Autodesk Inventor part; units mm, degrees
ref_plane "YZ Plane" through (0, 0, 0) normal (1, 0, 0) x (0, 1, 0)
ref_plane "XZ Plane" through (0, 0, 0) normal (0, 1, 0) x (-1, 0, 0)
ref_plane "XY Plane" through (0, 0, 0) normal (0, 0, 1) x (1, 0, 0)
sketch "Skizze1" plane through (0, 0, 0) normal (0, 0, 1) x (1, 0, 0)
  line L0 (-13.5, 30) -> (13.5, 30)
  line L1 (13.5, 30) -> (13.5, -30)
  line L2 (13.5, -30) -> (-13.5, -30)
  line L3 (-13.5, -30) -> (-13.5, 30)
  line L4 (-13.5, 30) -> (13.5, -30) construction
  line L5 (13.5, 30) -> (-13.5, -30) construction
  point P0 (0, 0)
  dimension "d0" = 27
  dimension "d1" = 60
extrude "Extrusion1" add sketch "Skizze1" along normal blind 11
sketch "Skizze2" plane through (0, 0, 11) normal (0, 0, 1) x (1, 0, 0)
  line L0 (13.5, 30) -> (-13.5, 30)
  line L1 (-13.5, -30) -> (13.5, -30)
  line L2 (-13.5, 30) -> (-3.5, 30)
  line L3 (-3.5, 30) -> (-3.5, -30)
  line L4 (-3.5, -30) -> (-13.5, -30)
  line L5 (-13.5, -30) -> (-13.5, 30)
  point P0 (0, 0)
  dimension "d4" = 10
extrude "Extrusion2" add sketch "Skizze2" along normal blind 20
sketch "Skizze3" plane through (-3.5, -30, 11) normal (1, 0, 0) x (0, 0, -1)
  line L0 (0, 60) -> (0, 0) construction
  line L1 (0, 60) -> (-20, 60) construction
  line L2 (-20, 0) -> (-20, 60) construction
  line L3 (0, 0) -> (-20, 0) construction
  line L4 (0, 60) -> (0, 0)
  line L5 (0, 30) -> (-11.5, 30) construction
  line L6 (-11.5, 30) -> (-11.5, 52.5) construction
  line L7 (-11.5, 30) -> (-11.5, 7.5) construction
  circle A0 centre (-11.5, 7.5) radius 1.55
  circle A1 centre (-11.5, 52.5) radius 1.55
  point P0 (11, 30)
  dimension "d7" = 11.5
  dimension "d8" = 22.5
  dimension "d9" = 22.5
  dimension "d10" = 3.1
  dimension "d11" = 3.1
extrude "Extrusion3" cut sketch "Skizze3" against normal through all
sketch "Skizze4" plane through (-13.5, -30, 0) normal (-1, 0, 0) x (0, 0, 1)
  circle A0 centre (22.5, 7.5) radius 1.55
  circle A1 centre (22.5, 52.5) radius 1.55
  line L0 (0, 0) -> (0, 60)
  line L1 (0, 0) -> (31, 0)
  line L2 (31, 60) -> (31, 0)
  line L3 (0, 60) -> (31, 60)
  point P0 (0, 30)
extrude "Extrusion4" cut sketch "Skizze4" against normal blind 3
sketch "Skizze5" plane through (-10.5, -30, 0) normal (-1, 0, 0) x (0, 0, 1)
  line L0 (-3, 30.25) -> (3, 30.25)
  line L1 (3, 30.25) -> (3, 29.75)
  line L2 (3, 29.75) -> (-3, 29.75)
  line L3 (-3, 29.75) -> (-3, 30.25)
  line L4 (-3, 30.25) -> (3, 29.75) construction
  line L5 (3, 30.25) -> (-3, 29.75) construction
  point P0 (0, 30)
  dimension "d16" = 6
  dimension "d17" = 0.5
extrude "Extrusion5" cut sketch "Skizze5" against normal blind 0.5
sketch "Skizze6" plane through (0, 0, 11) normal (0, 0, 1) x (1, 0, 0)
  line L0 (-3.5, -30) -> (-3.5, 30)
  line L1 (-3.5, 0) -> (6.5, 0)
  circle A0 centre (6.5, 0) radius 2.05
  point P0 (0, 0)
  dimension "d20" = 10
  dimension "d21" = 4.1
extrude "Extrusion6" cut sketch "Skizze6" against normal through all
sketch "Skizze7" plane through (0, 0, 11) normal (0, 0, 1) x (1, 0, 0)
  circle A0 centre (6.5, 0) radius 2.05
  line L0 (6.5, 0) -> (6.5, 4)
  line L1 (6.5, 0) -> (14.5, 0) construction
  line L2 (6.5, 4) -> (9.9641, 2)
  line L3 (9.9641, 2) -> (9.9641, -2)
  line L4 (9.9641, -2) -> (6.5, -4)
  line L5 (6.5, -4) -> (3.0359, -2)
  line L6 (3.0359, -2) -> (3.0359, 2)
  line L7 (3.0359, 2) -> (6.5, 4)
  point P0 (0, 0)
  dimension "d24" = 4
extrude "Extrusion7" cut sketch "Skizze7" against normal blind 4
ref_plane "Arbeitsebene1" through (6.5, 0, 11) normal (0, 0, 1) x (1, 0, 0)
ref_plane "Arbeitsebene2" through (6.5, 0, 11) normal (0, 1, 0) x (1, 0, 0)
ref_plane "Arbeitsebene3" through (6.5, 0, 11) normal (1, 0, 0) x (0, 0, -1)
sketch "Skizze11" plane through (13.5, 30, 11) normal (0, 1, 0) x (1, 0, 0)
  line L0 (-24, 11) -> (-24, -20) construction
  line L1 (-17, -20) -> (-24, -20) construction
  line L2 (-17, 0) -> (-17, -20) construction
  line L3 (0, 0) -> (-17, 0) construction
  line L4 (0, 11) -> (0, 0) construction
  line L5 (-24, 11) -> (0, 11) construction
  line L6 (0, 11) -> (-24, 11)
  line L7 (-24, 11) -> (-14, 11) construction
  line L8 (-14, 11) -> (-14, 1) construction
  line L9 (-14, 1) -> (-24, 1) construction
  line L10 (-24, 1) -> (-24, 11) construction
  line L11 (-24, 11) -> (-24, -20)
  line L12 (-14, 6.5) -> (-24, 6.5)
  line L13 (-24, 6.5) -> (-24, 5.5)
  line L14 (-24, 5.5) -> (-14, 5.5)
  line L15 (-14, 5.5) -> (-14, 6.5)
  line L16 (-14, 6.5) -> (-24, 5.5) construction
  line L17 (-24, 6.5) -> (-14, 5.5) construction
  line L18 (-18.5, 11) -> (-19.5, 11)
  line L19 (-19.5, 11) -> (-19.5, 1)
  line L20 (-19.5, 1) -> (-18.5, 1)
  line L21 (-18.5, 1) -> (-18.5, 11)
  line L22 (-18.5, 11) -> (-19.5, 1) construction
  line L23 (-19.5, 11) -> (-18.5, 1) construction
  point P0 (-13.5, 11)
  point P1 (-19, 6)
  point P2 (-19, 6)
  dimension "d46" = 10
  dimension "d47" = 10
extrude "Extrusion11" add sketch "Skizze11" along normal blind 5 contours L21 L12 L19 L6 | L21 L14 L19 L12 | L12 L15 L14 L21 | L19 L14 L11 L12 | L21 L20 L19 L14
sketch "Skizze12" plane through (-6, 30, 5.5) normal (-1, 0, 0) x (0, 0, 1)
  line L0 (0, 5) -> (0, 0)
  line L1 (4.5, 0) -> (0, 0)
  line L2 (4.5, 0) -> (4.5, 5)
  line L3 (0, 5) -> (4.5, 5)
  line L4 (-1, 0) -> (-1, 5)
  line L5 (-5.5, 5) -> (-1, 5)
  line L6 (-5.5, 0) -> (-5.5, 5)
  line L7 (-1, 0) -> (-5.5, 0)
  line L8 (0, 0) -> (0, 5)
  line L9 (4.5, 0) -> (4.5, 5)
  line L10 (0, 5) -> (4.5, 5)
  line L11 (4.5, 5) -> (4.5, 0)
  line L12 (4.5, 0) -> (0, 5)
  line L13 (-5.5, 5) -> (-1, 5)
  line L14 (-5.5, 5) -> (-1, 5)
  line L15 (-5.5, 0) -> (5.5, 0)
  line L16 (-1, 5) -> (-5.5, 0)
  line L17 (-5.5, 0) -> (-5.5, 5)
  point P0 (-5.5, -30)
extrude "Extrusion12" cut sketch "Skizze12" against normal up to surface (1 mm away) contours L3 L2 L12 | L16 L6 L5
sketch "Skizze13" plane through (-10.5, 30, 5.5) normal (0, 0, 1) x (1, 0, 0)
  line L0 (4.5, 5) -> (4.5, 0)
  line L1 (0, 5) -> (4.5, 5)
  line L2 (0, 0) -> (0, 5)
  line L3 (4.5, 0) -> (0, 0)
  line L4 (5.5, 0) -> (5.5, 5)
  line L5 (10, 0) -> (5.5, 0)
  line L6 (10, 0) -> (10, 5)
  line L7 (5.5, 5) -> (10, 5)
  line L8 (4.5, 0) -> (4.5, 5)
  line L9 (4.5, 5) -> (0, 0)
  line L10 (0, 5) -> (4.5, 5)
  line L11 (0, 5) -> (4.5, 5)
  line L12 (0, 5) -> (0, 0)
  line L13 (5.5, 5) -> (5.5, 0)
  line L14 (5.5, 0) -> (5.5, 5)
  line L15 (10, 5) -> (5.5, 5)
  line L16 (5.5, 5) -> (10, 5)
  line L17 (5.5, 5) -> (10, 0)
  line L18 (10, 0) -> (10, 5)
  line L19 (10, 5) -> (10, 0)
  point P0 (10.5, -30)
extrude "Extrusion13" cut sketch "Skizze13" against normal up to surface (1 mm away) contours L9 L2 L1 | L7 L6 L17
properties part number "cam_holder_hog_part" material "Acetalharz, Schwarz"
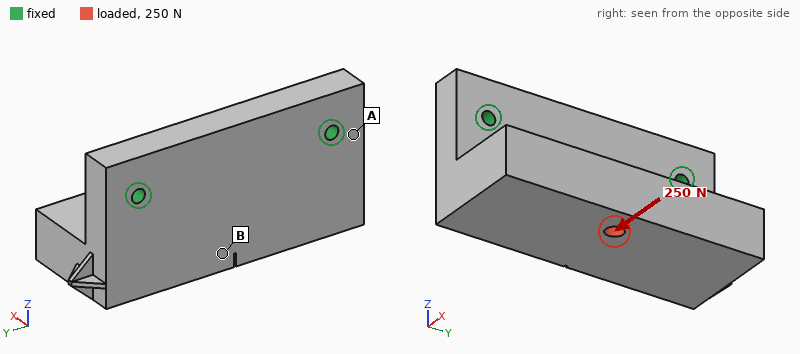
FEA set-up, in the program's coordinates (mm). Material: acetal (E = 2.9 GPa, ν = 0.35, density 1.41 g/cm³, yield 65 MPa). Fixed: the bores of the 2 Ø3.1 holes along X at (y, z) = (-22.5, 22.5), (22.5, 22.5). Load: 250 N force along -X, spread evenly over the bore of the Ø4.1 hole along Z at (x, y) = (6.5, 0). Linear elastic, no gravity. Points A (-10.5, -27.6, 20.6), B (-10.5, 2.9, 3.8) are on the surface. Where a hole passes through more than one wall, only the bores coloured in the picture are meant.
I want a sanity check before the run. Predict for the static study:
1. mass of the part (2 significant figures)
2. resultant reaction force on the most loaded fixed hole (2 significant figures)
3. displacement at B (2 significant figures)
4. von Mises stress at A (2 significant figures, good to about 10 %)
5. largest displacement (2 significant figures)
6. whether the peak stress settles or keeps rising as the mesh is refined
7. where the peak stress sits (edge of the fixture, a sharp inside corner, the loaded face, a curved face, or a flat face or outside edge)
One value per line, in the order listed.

34 g
130 N
0.24 mm
8.0 MPa
0.42 mm
keeps rising
edge of the fixture
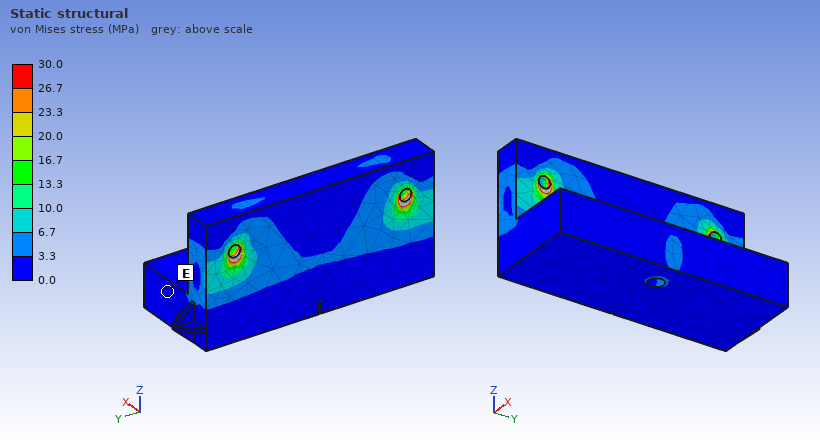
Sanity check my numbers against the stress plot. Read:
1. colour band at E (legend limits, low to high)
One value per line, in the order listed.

0.0 to 3.3 MPa
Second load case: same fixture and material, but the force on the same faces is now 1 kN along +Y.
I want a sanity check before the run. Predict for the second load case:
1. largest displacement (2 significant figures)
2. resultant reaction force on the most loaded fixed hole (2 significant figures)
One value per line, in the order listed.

0.26 mm
710 N
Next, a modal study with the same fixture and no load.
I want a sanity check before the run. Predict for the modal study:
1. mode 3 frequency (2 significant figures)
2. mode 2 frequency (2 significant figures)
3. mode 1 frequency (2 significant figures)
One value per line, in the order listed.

3300 Hz
2200 Hz
990 Hz
